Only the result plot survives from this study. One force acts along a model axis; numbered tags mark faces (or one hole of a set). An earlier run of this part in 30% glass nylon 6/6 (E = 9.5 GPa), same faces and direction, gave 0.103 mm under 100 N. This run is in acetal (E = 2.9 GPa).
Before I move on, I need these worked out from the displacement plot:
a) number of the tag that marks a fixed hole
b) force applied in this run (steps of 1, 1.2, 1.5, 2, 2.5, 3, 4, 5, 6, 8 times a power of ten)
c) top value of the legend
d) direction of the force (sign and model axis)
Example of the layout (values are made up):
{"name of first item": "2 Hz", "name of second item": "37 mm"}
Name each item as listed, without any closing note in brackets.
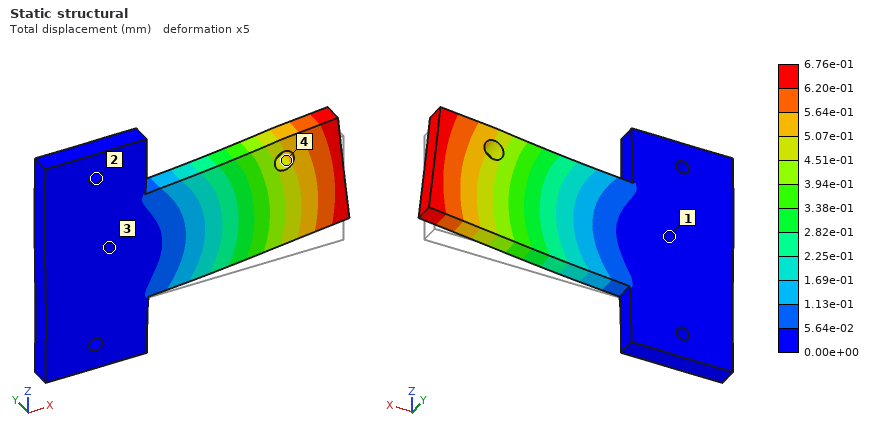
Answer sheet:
{"number of the tag that marks a fixed hole": "2", "force applied in this run": "200 N", "top value of the legend": "6.76e-01 mm", "direction of the force": "+Z"}
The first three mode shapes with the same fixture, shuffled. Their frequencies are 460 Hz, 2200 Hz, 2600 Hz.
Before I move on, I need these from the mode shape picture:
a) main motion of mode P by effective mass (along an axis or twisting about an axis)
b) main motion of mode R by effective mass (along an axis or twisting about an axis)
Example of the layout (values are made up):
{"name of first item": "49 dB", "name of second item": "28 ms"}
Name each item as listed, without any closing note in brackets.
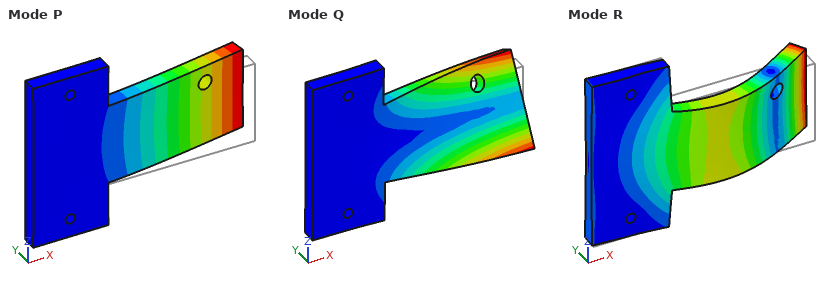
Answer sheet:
{"main motion of mode P by effective mass": "along Y", "main motion of mode R by effective mass": "along Y"}
